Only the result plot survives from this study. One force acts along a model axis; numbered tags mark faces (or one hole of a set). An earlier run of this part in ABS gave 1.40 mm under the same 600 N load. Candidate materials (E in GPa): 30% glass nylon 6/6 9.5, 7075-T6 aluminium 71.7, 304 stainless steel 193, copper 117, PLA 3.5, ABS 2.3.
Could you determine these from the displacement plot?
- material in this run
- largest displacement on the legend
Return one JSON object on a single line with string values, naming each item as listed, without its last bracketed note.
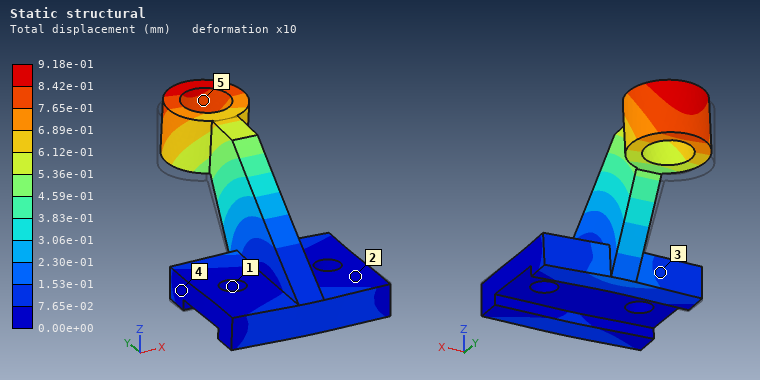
{"material in this run": "PLA", "largest displacement on the legend": "9.18e-01 mm"}
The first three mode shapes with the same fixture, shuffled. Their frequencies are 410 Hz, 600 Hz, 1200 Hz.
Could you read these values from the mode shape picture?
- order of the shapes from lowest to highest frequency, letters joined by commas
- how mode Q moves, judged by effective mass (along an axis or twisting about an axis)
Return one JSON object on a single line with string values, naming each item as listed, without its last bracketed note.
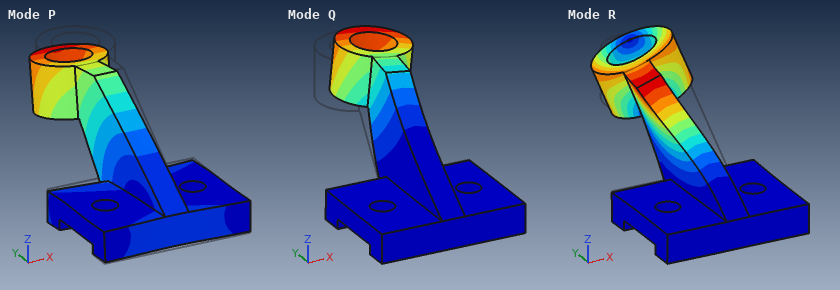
{"order of the shapes from lowest to highest frequency, letters joined by commas": "Q, P, R", "how mode Q moves, judged by effective mass": "along X"}
